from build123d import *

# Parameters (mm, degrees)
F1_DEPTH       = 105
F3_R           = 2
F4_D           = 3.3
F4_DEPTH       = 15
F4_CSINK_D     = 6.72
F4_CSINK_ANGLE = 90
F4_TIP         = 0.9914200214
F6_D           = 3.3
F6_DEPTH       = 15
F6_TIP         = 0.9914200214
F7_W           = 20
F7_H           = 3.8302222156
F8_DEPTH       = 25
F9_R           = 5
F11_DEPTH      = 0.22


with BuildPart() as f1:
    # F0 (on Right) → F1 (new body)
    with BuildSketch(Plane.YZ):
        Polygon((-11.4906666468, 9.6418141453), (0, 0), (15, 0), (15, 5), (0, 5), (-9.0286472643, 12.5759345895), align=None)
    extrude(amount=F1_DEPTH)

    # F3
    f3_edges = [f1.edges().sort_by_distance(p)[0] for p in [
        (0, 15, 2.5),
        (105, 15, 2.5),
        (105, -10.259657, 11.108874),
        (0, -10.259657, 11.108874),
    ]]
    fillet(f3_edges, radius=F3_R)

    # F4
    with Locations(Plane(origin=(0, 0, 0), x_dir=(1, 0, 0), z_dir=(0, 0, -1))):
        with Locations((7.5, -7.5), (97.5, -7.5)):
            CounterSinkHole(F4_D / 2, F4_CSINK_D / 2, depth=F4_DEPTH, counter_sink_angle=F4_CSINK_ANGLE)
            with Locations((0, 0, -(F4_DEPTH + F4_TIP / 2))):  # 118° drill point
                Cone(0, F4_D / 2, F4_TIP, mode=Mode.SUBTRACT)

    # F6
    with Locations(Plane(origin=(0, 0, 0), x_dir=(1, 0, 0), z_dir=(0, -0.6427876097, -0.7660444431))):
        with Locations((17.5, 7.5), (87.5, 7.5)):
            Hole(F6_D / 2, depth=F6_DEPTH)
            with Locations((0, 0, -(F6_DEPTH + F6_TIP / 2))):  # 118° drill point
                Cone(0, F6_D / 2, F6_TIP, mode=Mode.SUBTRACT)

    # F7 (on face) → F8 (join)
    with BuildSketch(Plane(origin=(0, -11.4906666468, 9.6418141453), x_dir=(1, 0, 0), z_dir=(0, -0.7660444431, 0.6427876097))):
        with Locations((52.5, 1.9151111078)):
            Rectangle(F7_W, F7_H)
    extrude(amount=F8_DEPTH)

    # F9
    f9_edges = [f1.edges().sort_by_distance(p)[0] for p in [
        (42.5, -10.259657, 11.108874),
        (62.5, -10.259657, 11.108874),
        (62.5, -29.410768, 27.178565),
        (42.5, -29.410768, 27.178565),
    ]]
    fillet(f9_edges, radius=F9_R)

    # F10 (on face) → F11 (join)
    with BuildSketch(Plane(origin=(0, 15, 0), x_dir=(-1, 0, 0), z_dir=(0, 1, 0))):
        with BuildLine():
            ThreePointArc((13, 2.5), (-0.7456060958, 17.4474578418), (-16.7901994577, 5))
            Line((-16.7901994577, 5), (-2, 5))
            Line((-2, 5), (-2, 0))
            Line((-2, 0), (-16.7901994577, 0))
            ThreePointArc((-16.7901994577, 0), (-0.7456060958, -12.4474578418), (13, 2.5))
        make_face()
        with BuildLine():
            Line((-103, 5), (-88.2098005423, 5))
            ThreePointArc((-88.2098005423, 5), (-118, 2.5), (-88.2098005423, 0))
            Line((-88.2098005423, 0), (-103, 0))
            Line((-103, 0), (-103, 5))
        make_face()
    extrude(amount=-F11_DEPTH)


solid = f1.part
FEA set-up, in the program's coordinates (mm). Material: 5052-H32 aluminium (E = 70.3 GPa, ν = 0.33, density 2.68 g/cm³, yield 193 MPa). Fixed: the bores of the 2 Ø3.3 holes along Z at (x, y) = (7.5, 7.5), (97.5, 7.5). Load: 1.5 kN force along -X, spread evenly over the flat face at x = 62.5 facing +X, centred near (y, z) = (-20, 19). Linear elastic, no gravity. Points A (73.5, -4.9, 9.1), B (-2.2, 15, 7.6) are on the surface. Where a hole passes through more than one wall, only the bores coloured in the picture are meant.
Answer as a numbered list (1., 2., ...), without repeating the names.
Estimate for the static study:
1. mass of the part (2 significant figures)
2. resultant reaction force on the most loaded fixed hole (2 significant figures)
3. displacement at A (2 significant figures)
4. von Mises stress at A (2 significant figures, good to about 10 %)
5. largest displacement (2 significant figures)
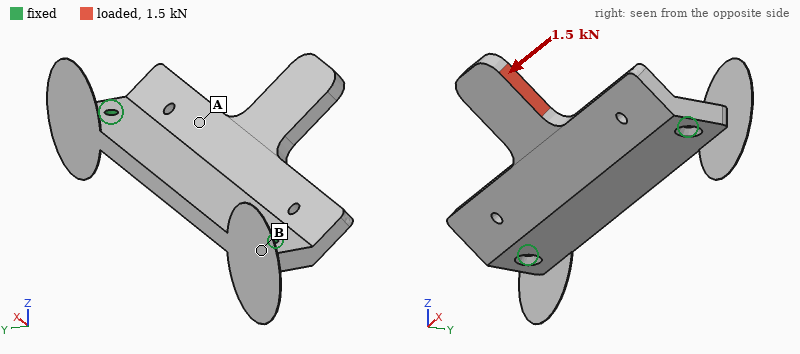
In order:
1. 41 g
2. 920 N
3. 26 µm
4. 37 MPa
5. 75 µm
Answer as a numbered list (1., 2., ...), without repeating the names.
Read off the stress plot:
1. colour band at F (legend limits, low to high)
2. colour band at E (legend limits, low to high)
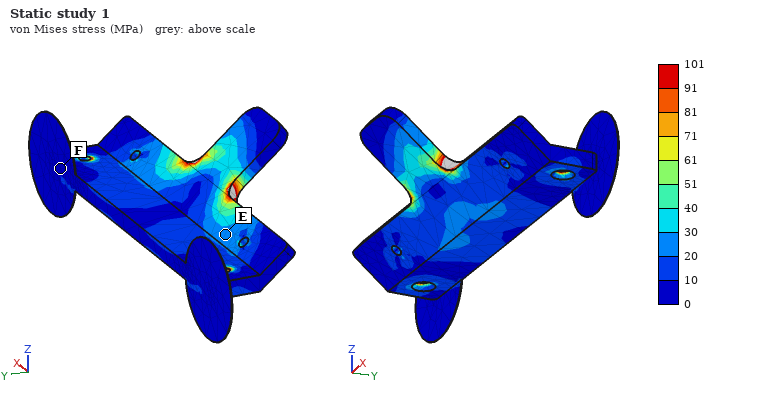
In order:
1. 0 to 10 MPa
2. 20 to 30 MPa
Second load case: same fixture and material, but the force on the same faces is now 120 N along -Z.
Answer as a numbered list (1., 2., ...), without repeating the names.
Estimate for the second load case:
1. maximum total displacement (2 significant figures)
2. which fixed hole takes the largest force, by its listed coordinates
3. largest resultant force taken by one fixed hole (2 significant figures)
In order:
1. 0.22 mm
2. (97.5, 7.5)
3. 78 N
